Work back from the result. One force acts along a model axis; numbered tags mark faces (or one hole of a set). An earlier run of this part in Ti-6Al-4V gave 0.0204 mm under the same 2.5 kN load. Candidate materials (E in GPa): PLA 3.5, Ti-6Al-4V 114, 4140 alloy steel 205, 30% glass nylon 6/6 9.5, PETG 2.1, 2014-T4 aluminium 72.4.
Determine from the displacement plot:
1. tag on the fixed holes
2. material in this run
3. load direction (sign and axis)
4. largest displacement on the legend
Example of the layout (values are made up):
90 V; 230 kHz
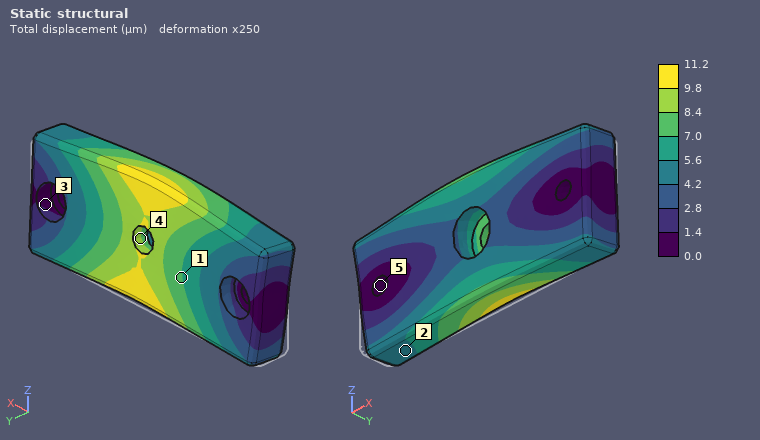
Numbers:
5; 4140 alloy steel; +Z; 11.2 µm
